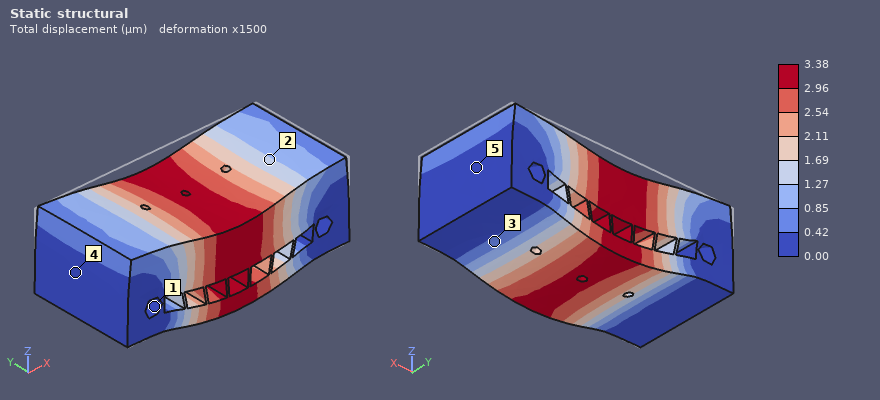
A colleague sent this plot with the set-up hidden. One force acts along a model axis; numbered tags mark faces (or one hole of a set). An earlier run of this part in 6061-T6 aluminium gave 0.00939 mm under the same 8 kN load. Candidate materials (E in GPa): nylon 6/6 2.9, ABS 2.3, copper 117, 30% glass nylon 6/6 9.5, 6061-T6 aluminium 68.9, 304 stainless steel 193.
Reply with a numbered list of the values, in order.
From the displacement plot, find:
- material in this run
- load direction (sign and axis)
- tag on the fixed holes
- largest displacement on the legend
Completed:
1. 304 stainless steel
2. -Z
3. 1
4. 3.38 µm
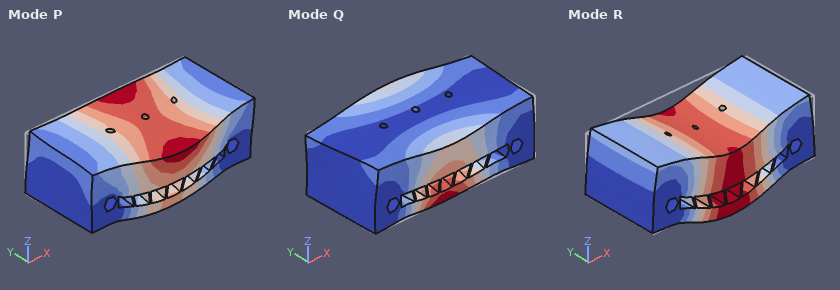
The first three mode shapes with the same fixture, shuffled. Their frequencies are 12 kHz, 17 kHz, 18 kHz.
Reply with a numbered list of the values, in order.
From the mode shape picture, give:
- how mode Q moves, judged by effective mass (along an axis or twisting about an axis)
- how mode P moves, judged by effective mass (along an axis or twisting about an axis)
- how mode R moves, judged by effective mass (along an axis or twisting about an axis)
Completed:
1. along Y
2. along Y
3. along Z
